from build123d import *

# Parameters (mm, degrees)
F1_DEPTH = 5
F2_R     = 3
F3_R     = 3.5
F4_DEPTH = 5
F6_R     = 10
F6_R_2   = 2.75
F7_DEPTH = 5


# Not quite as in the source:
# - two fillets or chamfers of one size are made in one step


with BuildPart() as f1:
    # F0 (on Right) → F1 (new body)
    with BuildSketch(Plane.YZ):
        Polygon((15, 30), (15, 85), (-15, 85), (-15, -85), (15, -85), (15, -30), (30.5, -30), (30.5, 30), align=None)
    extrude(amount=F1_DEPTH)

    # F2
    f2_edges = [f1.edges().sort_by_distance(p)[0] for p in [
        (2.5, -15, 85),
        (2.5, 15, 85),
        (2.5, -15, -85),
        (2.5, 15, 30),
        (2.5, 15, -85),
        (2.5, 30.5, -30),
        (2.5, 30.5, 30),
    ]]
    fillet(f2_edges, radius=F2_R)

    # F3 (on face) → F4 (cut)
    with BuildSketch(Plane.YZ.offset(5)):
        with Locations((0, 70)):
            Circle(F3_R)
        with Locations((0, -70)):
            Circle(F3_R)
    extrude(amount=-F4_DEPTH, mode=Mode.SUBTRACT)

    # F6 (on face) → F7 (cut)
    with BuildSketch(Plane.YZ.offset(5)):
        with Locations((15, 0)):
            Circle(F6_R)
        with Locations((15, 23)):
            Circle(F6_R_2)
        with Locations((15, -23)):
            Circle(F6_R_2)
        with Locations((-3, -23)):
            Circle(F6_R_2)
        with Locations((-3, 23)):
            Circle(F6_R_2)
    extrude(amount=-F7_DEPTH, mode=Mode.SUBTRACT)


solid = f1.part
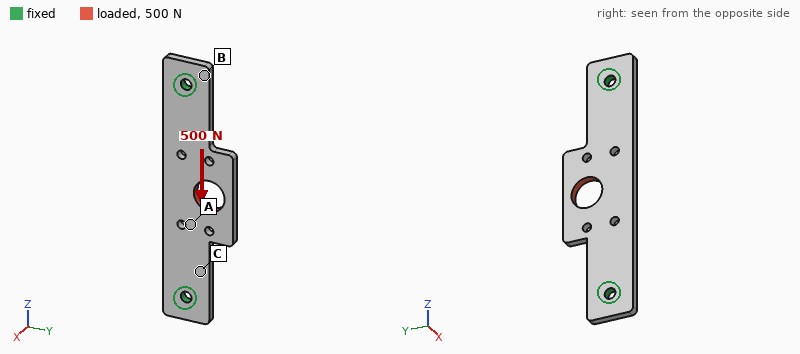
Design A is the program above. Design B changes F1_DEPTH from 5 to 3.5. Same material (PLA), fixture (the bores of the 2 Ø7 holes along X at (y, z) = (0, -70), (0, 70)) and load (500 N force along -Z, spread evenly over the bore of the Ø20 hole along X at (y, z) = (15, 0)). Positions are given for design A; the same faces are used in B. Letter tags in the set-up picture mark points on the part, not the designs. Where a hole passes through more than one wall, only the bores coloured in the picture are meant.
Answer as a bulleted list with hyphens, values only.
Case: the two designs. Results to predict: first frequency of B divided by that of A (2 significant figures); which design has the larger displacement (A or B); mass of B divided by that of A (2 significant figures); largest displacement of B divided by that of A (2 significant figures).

- 0.71
- B
- 0.70
- 1.4
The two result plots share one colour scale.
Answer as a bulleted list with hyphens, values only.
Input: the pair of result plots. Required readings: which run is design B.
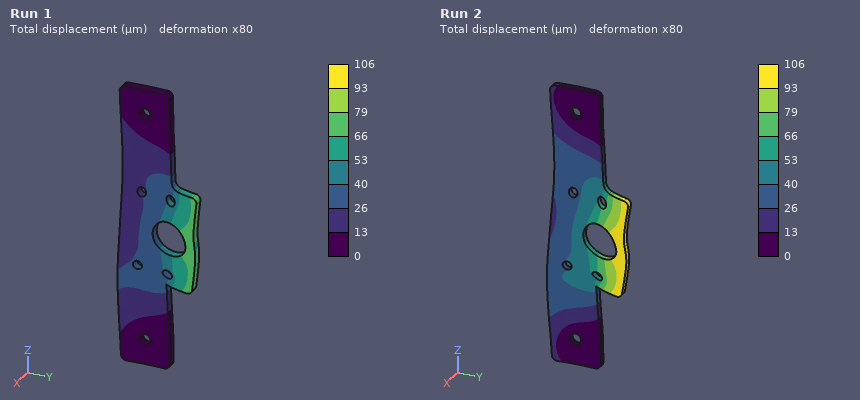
- Run 2
